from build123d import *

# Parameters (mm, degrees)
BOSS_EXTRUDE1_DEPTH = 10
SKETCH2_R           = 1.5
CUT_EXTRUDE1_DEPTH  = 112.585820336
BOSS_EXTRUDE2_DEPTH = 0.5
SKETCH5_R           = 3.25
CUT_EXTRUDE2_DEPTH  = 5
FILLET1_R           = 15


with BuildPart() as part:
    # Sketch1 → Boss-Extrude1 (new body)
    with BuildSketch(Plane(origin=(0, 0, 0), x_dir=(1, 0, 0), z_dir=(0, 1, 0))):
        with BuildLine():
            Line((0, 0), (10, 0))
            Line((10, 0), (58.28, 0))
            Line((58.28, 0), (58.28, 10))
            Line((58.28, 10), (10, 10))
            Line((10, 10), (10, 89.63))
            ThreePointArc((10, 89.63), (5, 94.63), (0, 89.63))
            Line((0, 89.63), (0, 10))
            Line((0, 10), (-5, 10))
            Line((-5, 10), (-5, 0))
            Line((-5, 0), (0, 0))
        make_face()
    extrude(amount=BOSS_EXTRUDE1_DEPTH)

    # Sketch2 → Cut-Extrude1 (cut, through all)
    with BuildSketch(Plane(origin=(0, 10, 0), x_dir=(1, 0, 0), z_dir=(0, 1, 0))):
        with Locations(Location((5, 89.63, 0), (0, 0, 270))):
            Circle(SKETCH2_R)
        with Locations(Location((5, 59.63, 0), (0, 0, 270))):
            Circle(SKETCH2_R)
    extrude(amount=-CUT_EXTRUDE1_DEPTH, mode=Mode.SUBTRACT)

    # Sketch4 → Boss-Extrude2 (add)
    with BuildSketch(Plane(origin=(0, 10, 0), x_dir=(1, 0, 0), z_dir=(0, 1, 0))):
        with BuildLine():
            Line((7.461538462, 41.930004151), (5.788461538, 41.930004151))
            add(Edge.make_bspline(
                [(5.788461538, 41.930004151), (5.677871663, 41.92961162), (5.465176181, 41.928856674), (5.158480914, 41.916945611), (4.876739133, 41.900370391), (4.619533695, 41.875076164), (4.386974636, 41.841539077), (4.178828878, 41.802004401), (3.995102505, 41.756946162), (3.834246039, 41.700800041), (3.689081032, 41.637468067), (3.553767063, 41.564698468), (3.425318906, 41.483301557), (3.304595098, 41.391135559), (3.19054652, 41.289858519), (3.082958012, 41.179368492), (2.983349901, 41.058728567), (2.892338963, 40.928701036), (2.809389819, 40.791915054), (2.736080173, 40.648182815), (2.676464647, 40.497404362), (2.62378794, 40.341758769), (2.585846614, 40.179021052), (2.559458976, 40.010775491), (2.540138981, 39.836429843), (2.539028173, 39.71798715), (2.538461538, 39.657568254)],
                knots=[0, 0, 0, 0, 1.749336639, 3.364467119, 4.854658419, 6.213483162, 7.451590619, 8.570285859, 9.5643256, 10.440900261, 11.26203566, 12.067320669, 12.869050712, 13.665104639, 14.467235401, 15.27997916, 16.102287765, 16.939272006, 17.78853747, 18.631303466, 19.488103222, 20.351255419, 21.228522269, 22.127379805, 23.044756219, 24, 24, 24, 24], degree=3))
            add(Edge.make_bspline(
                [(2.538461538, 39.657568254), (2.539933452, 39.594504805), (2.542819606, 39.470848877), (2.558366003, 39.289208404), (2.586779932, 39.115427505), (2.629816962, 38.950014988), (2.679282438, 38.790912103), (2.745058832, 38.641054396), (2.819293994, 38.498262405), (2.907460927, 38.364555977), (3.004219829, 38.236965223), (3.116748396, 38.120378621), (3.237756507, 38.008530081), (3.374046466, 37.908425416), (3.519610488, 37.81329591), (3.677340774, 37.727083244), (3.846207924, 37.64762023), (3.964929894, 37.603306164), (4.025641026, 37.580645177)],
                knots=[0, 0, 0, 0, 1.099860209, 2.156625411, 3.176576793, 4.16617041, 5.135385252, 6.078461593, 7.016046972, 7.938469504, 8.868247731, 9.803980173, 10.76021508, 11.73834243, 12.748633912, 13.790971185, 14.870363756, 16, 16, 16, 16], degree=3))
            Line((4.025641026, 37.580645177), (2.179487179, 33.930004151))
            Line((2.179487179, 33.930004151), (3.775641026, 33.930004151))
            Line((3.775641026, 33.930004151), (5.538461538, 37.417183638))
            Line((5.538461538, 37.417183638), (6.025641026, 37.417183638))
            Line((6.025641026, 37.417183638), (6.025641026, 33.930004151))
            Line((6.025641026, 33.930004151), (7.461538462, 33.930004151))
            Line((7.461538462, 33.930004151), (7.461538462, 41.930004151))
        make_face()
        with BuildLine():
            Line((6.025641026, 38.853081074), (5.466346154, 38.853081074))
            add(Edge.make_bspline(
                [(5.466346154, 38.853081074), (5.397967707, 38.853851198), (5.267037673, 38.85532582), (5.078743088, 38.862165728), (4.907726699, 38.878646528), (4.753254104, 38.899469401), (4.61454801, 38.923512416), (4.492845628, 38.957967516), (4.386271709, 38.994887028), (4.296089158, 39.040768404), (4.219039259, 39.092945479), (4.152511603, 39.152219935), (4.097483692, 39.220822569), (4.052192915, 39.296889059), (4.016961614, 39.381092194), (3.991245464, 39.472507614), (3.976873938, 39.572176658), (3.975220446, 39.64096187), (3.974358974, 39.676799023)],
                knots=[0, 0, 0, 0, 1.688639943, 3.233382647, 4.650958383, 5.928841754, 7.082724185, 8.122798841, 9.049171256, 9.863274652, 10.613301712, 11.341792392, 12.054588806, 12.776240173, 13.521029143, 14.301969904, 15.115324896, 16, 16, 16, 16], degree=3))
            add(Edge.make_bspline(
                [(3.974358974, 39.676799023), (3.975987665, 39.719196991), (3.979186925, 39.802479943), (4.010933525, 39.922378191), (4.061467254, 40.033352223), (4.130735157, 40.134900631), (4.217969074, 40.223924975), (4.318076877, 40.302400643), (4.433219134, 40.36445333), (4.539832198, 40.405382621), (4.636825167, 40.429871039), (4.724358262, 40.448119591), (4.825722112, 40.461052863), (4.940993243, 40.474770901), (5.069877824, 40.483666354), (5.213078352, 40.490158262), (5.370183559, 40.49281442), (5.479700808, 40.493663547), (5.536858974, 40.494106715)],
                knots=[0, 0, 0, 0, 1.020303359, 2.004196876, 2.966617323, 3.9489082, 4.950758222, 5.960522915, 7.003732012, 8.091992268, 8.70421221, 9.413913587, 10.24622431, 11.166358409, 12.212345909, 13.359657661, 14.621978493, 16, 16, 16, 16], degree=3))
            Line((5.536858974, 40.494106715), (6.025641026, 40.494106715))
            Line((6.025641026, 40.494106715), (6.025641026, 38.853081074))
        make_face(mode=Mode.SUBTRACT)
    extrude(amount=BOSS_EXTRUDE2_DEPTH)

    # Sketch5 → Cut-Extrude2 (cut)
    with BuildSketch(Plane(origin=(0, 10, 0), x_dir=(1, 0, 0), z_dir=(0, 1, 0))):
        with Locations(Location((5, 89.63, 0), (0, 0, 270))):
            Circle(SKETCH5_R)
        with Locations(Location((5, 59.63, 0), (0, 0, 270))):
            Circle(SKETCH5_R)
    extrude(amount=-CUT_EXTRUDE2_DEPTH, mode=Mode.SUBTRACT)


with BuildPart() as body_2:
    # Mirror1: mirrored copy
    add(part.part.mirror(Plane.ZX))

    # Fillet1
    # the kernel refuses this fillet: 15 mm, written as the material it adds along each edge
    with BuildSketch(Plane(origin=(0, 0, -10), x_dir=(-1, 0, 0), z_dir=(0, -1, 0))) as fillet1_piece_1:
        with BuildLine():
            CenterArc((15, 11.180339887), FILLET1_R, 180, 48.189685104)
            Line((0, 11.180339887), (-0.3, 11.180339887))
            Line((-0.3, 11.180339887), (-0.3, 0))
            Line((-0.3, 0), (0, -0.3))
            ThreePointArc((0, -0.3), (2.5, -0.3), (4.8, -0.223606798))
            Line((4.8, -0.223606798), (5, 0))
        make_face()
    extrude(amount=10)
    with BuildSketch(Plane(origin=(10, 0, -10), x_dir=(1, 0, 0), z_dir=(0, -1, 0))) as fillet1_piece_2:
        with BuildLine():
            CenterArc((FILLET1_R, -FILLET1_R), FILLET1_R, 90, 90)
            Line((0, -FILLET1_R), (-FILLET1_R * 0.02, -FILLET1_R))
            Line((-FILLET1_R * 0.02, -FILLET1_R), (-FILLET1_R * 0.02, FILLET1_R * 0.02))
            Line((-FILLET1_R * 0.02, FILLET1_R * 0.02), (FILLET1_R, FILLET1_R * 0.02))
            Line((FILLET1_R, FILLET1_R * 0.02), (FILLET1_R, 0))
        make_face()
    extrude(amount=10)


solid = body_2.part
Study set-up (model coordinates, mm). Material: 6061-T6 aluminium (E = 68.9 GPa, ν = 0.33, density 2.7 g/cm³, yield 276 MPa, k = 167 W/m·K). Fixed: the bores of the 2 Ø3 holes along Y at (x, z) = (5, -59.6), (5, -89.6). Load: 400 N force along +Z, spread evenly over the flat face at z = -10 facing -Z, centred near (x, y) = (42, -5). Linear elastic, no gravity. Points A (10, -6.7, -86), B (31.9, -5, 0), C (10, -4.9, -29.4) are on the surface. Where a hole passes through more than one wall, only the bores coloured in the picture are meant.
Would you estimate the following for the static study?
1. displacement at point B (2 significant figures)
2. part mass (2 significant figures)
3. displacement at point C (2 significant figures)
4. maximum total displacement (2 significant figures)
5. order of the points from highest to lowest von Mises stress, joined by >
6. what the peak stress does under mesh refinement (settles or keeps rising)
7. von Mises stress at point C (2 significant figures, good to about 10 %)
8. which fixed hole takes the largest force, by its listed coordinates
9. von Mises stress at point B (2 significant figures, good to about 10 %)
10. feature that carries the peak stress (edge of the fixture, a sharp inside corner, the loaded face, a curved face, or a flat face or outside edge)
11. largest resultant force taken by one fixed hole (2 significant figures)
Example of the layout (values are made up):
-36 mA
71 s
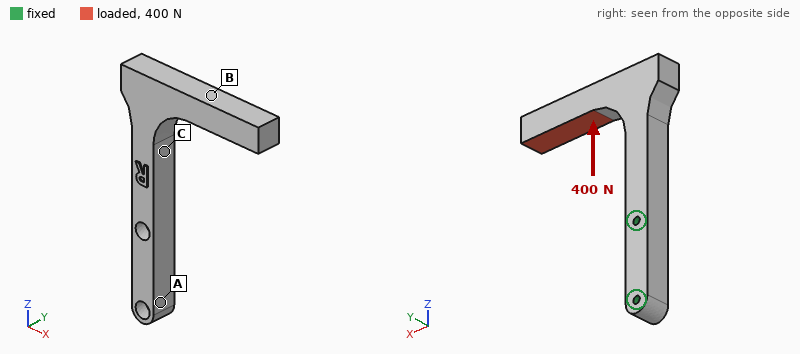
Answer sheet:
0.66 mm
40 g
0.18 mm
0.96 mm
C > B > A
keeps rising
92 MPa
(5, -59.6)
25 MPa
edge of the fixture
470 N
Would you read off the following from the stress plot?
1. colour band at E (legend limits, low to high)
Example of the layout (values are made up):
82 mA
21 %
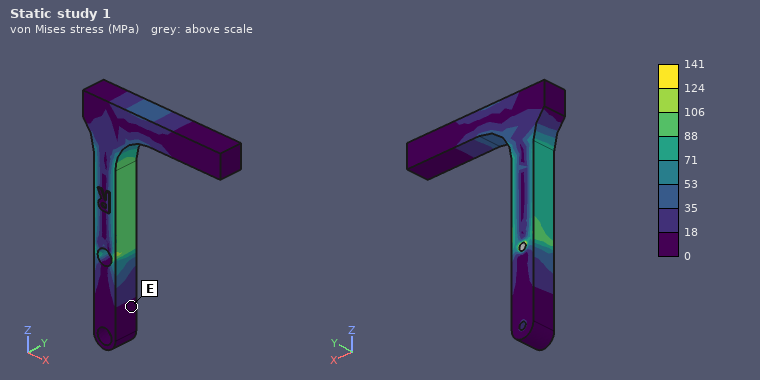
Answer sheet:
0 to 18 MPa
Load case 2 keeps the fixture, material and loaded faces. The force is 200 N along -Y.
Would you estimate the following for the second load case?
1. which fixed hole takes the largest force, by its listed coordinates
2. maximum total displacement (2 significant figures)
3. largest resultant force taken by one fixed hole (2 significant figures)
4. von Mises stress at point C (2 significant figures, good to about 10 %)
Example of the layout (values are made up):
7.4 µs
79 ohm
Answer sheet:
(5, -59.6)
0.88 mm
550 N
66 MPa
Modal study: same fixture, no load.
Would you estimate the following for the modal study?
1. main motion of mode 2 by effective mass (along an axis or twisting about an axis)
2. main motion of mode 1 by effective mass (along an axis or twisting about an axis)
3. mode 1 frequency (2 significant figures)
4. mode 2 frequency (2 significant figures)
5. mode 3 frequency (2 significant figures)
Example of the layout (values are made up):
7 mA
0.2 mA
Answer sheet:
along X
along Y
770 Hz
810 Hz
1800 Hz
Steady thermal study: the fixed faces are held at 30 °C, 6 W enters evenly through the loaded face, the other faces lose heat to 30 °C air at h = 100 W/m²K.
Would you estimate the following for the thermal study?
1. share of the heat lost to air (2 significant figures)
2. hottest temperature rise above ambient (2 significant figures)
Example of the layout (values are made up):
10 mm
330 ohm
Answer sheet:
59 %
16 K
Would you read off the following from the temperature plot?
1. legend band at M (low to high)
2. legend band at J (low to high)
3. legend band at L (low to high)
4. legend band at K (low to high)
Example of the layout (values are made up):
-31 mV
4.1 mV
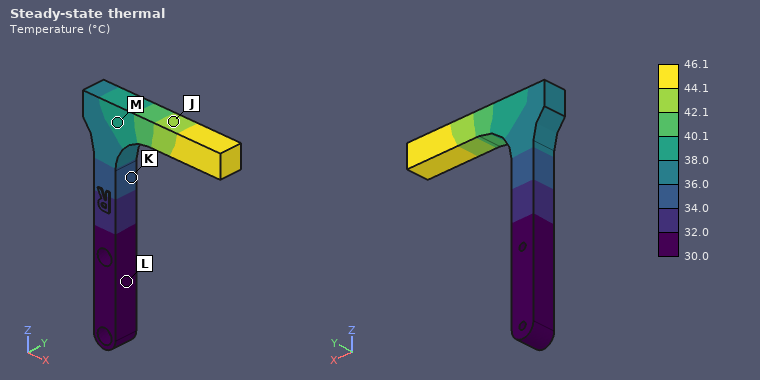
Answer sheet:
38.0 to 40.1 °C
42.1 to 44.1 °C
30.0 to 32.0 °C
34.0 to 36.0 °C
